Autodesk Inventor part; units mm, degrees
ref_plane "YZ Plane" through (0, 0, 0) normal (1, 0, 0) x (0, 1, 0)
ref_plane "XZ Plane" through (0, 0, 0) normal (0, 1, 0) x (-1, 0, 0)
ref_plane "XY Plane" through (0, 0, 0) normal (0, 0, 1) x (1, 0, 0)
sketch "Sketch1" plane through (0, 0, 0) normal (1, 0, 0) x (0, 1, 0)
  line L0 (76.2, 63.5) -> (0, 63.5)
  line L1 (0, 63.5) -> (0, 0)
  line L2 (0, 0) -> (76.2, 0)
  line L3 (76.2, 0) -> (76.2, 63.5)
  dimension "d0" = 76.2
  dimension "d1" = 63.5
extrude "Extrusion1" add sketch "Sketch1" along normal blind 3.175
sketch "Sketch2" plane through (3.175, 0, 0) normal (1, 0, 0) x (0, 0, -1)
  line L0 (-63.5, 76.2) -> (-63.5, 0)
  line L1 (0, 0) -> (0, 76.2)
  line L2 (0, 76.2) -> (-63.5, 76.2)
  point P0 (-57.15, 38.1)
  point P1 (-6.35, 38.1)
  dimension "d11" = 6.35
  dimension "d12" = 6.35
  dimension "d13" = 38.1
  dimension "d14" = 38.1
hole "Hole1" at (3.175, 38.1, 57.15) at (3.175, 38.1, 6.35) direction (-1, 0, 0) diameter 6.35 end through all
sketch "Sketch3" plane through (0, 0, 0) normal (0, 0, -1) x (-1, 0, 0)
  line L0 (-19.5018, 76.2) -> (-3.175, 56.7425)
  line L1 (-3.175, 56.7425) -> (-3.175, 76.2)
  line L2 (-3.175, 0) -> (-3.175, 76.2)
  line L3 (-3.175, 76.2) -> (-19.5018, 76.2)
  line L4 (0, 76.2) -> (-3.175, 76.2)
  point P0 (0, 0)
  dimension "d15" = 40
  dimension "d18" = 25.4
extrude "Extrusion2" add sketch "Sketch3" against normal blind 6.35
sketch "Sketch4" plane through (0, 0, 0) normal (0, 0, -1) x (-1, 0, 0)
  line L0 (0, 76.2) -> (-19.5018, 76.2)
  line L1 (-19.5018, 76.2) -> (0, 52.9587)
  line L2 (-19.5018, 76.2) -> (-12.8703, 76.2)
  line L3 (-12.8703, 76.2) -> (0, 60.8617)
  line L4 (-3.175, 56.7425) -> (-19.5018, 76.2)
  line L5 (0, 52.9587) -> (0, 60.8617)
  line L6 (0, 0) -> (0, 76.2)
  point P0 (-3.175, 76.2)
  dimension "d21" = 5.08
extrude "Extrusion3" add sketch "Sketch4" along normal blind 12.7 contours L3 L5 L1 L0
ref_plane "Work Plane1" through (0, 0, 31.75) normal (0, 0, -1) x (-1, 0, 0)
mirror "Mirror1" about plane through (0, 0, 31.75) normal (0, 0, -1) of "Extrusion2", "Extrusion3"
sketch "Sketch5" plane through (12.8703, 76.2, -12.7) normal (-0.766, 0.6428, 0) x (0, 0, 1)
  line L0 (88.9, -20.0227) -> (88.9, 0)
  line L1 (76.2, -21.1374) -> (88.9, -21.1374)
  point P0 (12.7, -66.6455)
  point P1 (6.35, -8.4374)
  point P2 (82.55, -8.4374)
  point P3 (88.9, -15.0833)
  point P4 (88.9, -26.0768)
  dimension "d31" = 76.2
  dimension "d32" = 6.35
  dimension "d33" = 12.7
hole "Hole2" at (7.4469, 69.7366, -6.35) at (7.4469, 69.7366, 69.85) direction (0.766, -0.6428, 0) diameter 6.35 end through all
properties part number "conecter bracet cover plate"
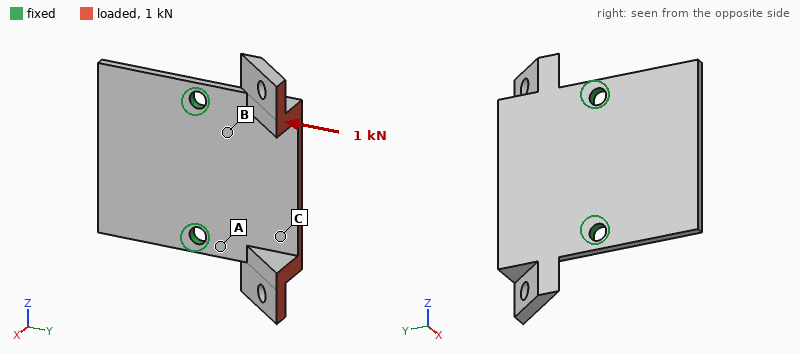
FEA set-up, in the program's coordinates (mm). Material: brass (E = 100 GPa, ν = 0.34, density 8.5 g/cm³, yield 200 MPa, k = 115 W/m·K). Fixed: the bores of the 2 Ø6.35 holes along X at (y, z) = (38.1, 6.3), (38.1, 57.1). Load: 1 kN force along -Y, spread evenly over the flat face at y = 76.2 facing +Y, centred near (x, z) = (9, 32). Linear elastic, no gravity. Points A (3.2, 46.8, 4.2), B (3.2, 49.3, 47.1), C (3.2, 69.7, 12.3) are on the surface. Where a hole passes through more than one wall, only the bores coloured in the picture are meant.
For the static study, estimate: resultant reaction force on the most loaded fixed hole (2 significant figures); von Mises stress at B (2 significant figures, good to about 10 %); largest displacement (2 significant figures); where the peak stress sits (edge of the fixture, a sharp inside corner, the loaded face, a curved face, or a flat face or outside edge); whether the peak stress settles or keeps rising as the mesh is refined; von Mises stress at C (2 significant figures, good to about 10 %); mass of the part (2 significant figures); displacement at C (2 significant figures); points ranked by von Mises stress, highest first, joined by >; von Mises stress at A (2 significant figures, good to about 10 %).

500 N
64 MPa
0.37 mm
edge of the fixture
keeps rising
24 MPa
170 g
0.22 mm
A > B > C
100 MPa
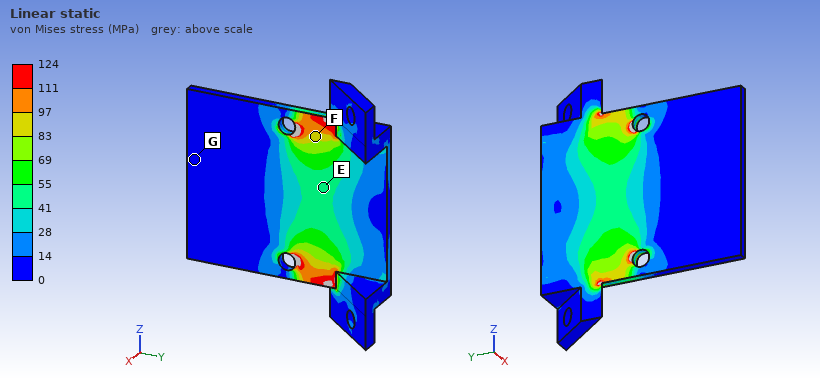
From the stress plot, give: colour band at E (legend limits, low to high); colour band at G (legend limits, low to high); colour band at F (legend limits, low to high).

41 to 55 MPa
0 to 14 MPa
83 to 97 MPa
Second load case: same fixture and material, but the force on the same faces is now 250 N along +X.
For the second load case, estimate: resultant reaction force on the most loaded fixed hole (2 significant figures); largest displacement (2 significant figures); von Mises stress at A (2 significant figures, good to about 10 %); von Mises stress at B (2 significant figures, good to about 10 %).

130 N
0.32 mm
89 MPa
54 MPa
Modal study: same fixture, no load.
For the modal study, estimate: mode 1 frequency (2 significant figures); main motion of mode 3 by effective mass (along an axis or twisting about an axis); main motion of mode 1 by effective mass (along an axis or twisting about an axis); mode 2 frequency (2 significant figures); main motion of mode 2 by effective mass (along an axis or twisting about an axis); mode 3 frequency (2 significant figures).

750 Hz
along X
along X
980 Hz
twisting about Y
1200 Hz
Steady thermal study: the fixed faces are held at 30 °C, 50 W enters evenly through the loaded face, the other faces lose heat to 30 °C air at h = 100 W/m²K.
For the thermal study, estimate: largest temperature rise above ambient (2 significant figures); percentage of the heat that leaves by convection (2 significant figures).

59 K
51 %
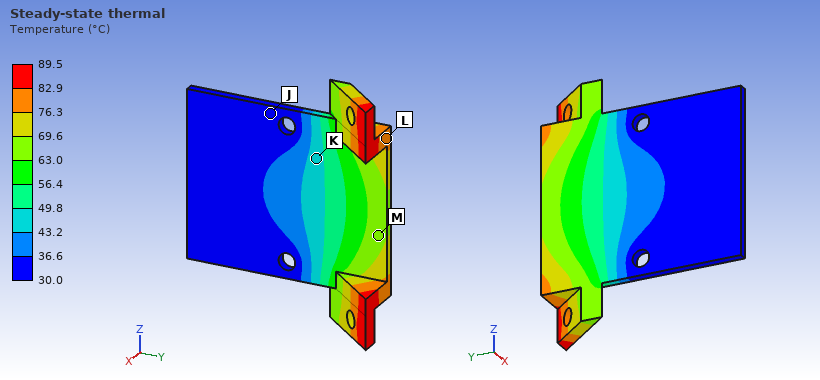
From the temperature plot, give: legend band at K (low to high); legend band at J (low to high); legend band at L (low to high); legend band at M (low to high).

43.2 to 49.8 °C
30.0 to 36.6 °C
76.3 to 82.9 °C
63.0 to 69.6 °C
